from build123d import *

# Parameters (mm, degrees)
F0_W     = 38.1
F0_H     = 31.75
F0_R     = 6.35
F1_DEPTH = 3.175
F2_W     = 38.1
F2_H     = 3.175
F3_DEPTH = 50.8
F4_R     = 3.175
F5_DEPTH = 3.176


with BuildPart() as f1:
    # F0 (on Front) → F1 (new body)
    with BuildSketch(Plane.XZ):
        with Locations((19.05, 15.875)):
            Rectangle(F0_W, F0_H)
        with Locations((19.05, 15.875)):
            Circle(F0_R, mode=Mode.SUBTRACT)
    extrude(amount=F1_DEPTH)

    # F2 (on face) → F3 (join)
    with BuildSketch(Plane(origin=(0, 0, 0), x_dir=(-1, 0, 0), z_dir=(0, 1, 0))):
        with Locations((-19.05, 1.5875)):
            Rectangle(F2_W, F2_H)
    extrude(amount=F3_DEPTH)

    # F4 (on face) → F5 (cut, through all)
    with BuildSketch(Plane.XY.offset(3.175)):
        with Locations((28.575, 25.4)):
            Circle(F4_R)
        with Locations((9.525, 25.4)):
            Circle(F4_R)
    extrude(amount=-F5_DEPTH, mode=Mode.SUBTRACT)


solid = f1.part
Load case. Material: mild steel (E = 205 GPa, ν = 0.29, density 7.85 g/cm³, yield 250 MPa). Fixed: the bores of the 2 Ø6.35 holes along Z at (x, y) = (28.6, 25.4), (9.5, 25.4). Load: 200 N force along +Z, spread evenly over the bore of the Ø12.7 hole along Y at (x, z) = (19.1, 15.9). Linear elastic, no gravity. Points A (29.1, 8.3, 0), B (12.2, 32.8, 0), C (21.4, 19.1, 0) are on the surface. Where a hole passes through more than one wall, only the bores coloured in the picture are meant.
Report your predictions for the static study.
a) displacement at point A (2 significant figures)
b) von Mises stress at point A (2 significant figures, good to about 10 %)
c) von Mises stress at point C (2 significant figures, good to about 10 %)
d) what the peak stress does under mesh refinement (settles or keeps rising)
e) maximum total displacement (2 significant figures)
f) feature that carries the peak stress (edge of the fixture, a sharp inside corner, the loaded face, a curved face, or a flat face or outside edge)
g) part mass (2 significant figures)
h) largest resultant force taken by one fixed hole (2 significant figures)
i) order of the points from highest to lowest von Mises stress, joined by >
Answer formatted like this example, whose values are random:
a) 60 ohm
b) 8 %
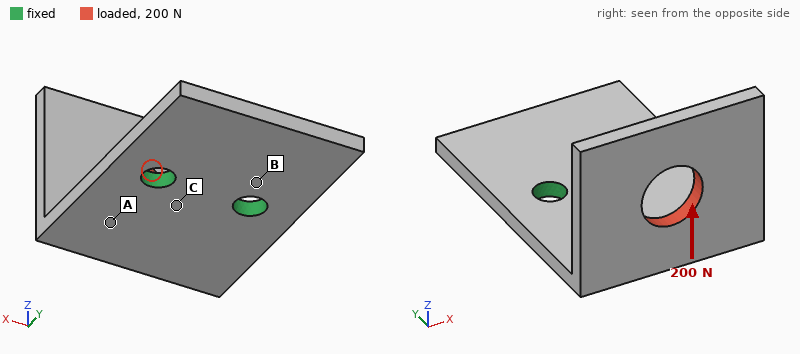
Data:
a) 0.023 mm
b) 28 MPa
c) 52 MPa
d) keeps rising
e) 0.10 mm
f) edge of the fixture
g) 74 g
h) 100 N
i) C > A > B
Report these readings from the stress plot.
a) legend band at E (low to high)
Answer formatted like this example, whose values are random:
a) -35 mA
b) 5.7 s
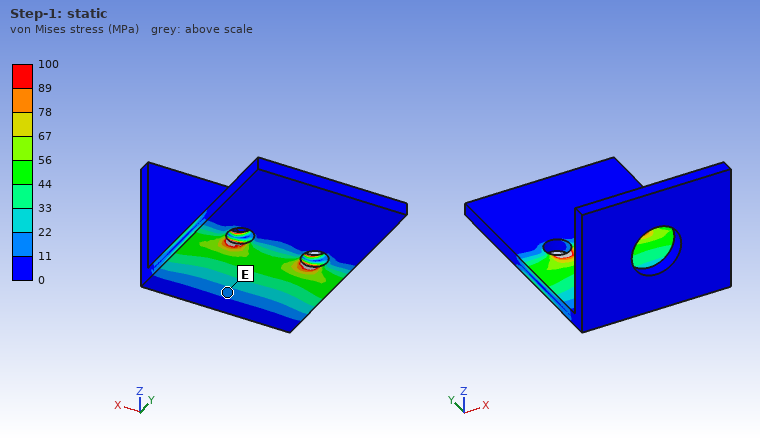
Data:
a) 11 to 22 MPa
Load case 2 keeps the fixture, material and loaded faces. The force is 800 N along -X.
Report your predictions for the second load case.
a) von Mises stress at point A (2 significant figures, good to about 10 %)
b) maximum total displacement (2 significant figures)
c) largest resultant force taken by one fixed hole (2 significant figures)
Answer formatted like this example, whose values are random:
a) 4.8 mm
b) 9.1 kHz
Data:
a) 89 MPa
b) 0.19 mm
c) 1.1 kN
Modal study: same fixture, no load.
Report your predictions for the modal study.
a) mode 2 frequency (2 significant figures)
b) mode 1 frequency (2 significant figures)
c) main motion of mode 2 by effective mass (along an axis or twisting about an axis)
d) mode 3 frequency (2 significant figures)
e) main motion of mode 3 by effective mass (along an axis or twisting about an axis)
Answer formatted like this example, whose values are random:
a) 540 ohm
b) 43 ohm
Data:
a) 2100 Hz
b) 1200 Hz
c) along X
d) 3200 Hz
e) along Z
